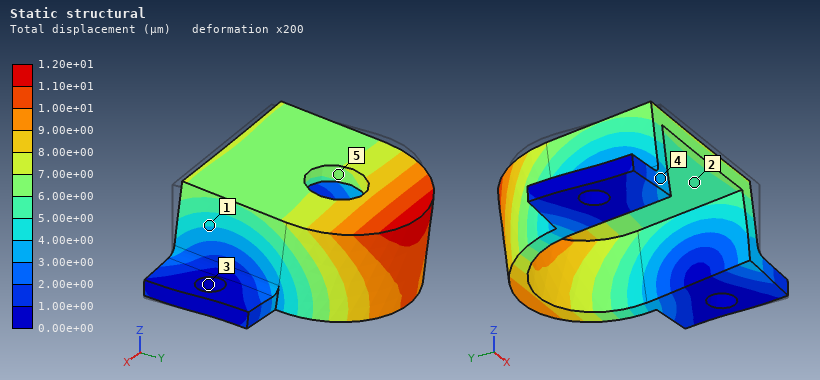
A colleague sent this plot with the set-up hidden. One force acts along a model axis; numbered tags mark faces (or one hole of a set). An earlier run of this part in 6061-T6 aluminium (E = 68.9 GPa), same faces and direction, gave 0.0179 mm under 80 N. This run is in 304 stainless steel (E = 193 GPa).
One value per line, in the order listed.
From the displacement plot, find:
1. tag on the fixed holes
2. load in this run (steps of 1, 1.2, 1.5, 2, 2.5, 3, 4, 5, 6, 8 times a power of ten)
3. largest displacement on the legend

3
150 N
1.20e+01 µm
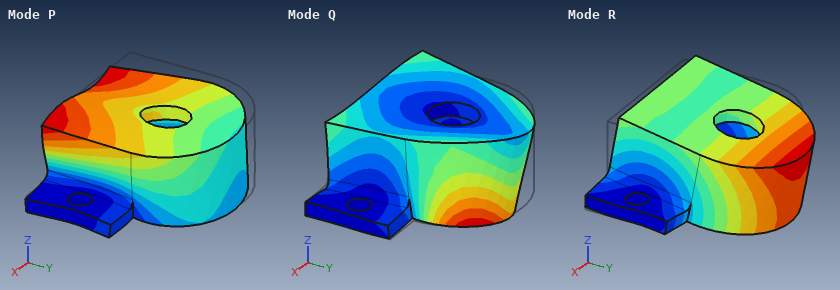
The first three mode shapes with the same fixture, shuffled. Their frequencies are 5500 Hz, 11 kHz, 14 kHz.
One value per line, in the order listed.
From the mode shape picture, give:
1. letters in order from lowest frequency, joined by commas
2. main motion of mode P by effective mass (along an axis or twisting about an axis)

R, P, Q
along X
